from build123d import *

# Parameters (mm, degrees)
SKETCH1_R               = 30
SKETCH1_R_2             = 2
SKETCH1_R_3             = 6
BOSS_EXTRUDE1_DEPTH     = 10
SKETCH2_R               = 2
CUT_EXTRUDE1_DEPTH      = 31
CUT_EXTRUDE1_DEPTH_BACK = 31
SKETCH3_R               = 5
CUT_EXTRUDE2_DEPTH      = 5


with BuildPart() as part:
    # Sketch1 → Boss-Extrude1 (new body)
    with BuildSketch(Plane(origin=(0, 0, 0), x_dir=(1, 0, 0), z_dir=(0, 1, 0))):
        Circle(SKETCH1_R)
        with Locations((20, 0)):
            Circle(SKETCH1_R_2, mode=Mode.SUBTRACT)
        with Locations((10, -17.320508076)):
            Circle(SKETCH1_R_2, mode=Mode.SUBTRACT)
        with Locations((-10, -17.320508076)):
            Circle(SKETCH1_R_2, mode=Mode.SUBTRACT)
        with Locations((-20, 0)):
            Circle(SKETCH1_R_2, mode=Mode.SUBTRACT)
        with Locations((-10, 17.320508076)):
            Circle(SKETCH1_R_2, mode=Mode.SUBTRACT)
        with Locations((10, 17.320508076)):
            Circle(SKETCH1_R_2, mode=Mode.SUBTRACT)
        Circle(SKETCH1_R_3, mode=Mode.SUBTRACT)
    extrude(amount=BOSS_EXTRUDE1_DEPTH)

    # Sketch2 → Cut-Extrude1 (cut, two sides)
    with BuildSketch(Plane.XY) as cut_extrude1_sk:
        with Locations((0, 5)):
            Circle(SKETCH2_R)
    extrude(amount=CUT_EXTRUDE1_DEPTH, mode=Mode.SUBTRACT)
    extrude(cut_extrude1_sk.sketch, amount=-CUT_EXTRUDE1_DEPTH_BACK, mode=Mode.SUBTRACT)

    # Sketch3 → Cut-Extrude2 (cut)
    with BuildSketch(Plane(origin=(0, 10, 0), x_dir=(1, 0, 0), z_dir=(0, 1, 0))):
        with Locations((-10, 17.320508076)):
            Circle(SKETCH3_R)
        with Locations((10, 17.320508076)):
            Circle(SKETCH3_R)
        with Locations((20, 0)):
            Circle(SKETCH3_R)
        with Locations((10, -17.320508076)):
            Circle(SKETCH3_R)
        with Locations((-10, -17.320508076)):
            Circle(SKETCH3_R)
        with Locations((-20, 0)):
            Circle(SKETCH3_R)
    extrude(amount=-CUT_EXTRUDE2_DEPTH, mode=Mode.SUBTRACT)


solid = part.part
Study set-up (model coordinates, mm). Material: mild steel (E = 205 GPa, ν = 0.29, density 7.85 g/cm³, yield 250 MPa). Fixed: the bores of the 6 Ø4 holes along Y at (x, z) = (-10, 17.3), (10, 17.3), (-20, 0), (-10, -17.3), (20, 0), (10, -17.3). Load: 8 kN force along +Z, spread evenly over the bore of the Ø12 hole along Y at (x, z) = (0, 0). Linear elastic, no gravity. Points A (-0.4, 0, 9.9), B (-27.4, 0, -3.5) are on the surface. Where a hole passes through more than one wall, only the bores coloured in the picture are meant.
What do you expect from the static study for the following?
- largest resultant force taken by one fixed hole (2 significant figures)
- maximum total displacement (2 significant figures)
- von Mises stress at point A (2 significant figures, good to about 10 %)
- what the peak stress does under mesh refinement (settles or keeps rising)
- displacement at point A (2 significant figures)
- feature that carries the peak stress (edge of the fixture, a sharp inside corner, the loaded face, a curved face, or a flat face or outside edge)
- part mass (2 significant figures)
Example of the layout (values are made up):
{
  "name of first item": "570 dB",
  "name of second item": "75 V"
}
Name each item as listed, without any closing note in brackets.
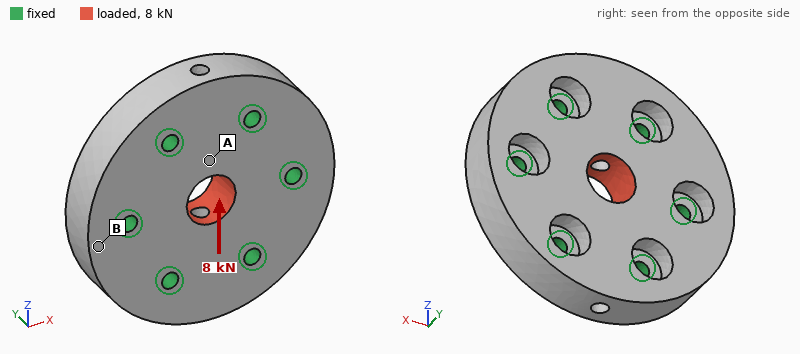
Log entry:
{
  "largest resultant force taken by one fixed hole": "1.7 kN",
  "maximum total displacement": "2.2 µm",
  "von Mises stress at point A": "19 MPa",
  "what the peak stress does under mesh refinement": "keeps rising",
  "displacement at point A": "1.2 µm",
  "feature that carries the peak stress": "edge of the fixture",
  "part mass": "190 g"
}
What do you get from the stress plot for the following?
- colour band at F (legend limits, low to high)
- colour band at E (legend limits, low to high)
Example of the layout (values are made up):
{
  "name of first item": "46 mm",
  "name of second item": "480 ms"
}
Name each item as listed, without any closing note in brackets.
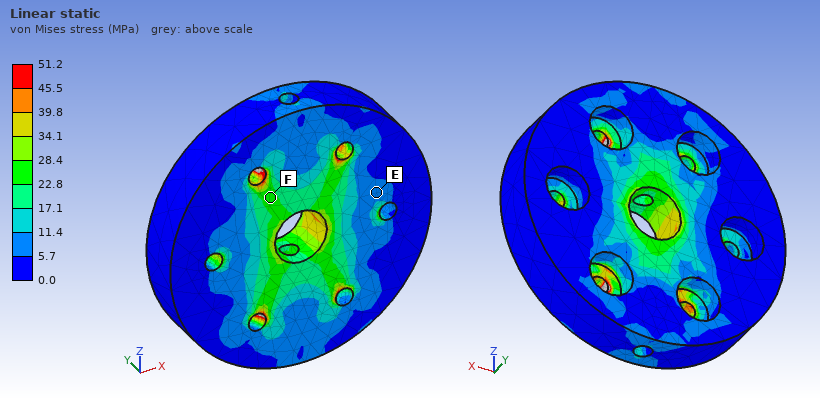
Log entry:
{
  "colour band at F": "22.8 to 28.4 MPa",
  "colour band at E": "5.7 to 11.4 MPa"
}
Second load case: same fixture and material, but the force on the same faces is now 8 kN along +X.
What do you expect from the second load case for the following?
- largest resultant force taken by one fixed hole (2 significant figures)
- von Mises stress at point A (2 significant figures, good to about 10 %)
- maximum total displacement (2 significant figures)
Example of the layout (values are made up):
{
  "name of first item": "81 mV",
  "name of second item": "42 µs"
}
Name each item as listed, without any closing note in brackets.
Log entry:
{
  "largest resultant force taken by one fixed hole": "1.9 kN",
  "von Mises stress at point A": "25 MPa",
  "maximum total displacement": "2.4 µm"
}
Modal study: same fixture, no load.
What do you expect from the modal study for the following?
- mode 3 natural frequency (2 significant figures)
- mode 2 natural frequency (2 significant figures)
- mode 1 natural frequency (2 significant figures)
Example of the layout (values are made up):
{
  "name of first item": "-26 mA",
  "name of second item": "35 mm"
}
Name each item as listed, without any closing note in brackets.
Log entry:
{
  "mode 3 natural frequency": "26 kHz",
  "mode 2 natural frequency": "26 kHz",
  "mode 1 natural frequency": "25 kHz"
}
